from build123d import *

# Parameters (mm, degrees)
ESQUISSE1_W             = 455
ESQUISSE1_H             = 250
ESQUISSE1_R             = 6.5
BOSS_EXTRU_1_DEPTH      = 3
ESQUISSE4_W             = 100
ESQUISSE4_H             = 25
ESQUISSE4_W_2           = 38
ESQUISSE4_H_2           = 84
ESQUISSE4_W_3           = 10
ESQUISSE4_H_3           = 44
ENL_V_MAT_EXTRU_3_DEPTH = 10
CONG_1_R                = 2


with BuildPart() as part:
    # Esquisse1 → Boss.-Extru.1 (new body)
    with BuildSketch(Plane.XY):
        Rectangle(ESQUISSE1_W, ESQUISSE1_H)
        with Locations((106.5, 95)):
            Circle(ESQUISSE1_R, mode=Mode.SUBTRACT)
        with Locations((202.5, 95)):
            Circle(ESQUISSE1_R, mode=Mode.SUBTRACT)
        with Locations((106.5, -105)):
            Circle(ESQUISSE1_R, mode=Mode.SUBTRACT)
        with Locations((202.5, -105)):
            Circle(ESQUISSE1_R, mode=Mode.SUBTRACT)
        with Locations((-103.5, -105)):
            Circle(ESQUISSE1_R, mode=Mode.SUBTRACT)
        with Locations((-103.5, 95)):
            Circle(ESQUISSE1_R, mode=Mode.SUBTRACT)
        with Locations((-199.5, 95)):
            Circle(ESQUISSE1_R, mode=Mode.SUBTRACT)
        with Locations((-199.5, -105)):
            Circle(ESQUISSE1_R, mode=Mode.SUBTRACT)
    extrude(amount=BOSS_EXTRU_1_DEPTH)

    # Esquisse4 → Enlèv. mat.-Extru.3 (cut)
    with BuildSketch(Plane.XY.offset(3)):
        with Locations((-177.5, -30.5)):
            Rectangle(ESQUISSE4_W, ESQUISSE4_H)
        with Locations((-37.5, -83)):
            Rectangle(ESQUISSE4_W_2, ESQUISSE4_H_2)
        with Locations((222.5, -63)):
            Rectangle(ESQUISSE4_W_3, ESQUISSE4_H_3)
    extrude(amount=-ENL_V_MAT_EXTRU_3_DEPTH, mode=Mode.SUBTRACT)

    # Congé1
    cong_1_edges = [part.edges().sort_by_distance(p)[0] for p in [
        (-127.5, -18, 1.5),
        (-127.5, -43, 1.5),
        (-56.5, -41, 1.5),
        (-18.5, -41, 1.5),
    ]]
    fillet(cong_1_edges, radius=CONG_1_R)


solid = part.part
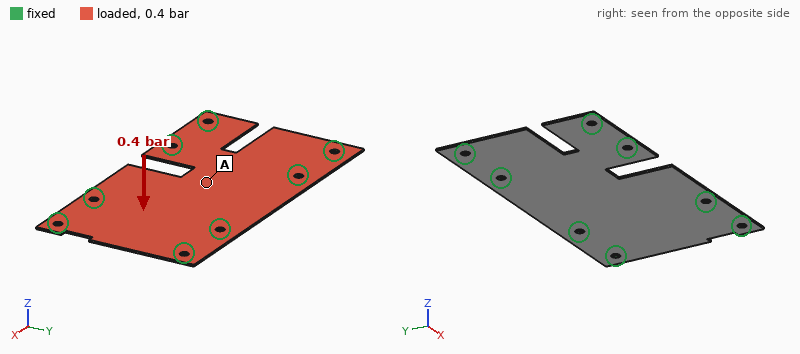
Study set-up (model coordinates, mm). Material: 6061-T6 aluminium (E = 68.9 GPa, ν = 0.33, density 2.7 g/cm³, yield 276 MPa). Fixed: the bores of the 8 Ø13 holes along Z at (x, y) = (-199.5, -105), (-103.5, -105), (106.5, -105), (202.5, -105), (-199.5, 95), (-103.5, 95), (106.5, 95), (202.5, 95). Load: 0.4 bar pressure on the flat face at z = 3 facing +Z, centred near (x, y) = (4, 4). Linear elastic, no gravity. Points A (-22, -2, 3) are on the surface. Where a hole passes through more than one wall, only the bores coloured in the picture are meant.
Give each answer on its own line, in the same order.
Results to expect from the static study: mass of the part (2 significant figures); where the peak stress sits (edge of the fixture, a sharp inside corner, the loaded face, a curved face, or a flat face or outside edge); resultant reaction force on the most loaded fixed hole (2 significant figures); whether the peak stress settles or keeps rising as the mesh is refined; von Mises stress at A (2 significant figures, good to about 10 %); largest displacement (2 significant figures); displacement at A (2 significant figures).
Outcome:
860 g
edge of the fixture
810 N
keeps rising
49 MPa
3.6 mm
2.8 mm
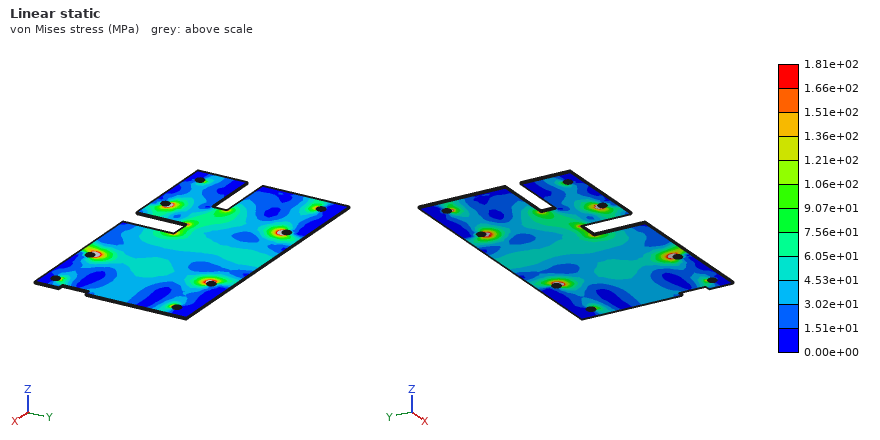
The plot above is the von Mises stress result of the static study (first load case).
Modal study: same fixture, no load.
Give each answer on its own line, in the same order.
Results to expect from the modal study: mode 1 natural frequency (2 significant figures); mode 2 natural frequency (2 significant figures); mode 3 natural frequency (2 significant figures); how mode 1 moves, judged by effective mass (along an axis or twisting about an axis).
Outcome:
250 Hz
310 Hz
350 Hz
along Z
